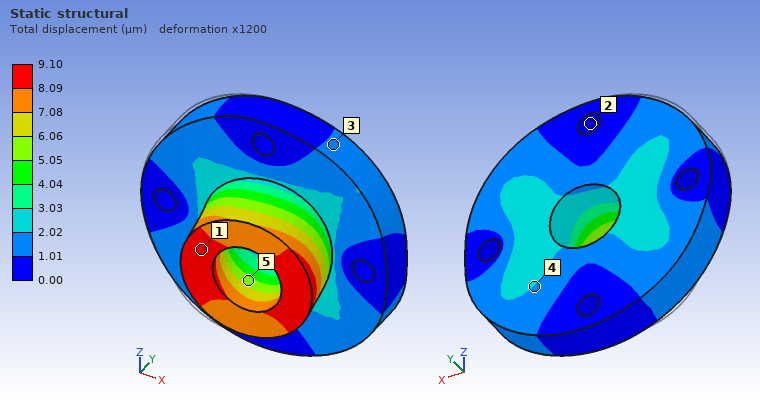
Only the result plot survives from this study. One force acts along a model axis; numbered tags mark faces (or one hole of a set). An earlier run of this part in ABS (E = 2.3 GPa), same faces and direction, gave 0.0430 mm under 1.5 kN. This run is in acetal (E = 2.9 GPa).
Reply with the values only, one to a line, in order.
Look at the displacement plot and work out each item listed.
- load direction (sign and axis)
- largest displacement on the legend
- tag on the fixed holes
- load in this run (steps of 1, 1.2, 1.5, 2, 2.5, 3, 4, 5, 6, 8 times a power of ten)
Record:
+X
9.10 µm
2
400 N
